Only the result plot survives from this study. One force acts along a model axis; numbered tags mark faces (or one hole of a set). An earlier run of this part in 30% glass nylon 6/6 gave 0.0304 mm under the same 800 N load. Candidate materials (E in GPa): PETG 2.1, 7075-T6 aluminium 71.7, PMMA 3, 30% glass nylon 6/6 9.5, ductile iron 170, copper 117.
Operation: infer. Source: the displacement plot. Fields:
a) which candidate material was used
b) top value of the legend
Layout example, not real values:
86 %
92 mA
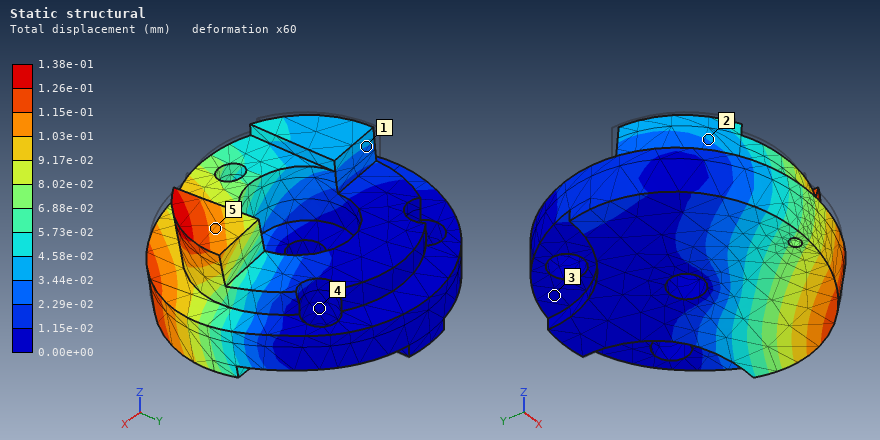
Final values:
PETG
1.38e-01 mm
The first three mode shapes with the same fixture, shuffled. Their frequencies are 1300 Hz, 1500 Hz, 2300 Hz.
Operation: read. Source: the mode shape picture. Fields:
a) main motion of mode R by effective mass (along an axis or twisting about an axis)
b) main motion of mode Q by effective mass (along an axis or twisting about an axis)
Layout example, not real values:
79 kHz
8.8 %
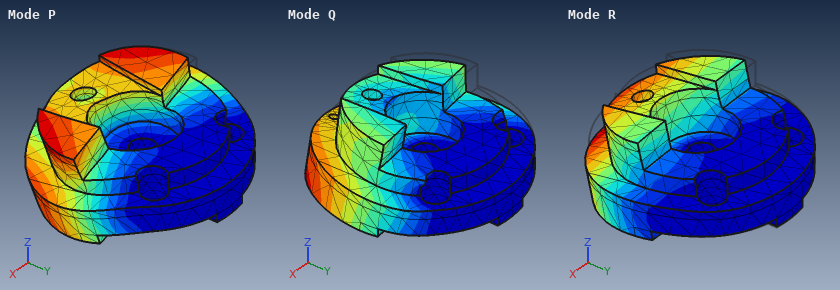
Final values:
along Z
along X
